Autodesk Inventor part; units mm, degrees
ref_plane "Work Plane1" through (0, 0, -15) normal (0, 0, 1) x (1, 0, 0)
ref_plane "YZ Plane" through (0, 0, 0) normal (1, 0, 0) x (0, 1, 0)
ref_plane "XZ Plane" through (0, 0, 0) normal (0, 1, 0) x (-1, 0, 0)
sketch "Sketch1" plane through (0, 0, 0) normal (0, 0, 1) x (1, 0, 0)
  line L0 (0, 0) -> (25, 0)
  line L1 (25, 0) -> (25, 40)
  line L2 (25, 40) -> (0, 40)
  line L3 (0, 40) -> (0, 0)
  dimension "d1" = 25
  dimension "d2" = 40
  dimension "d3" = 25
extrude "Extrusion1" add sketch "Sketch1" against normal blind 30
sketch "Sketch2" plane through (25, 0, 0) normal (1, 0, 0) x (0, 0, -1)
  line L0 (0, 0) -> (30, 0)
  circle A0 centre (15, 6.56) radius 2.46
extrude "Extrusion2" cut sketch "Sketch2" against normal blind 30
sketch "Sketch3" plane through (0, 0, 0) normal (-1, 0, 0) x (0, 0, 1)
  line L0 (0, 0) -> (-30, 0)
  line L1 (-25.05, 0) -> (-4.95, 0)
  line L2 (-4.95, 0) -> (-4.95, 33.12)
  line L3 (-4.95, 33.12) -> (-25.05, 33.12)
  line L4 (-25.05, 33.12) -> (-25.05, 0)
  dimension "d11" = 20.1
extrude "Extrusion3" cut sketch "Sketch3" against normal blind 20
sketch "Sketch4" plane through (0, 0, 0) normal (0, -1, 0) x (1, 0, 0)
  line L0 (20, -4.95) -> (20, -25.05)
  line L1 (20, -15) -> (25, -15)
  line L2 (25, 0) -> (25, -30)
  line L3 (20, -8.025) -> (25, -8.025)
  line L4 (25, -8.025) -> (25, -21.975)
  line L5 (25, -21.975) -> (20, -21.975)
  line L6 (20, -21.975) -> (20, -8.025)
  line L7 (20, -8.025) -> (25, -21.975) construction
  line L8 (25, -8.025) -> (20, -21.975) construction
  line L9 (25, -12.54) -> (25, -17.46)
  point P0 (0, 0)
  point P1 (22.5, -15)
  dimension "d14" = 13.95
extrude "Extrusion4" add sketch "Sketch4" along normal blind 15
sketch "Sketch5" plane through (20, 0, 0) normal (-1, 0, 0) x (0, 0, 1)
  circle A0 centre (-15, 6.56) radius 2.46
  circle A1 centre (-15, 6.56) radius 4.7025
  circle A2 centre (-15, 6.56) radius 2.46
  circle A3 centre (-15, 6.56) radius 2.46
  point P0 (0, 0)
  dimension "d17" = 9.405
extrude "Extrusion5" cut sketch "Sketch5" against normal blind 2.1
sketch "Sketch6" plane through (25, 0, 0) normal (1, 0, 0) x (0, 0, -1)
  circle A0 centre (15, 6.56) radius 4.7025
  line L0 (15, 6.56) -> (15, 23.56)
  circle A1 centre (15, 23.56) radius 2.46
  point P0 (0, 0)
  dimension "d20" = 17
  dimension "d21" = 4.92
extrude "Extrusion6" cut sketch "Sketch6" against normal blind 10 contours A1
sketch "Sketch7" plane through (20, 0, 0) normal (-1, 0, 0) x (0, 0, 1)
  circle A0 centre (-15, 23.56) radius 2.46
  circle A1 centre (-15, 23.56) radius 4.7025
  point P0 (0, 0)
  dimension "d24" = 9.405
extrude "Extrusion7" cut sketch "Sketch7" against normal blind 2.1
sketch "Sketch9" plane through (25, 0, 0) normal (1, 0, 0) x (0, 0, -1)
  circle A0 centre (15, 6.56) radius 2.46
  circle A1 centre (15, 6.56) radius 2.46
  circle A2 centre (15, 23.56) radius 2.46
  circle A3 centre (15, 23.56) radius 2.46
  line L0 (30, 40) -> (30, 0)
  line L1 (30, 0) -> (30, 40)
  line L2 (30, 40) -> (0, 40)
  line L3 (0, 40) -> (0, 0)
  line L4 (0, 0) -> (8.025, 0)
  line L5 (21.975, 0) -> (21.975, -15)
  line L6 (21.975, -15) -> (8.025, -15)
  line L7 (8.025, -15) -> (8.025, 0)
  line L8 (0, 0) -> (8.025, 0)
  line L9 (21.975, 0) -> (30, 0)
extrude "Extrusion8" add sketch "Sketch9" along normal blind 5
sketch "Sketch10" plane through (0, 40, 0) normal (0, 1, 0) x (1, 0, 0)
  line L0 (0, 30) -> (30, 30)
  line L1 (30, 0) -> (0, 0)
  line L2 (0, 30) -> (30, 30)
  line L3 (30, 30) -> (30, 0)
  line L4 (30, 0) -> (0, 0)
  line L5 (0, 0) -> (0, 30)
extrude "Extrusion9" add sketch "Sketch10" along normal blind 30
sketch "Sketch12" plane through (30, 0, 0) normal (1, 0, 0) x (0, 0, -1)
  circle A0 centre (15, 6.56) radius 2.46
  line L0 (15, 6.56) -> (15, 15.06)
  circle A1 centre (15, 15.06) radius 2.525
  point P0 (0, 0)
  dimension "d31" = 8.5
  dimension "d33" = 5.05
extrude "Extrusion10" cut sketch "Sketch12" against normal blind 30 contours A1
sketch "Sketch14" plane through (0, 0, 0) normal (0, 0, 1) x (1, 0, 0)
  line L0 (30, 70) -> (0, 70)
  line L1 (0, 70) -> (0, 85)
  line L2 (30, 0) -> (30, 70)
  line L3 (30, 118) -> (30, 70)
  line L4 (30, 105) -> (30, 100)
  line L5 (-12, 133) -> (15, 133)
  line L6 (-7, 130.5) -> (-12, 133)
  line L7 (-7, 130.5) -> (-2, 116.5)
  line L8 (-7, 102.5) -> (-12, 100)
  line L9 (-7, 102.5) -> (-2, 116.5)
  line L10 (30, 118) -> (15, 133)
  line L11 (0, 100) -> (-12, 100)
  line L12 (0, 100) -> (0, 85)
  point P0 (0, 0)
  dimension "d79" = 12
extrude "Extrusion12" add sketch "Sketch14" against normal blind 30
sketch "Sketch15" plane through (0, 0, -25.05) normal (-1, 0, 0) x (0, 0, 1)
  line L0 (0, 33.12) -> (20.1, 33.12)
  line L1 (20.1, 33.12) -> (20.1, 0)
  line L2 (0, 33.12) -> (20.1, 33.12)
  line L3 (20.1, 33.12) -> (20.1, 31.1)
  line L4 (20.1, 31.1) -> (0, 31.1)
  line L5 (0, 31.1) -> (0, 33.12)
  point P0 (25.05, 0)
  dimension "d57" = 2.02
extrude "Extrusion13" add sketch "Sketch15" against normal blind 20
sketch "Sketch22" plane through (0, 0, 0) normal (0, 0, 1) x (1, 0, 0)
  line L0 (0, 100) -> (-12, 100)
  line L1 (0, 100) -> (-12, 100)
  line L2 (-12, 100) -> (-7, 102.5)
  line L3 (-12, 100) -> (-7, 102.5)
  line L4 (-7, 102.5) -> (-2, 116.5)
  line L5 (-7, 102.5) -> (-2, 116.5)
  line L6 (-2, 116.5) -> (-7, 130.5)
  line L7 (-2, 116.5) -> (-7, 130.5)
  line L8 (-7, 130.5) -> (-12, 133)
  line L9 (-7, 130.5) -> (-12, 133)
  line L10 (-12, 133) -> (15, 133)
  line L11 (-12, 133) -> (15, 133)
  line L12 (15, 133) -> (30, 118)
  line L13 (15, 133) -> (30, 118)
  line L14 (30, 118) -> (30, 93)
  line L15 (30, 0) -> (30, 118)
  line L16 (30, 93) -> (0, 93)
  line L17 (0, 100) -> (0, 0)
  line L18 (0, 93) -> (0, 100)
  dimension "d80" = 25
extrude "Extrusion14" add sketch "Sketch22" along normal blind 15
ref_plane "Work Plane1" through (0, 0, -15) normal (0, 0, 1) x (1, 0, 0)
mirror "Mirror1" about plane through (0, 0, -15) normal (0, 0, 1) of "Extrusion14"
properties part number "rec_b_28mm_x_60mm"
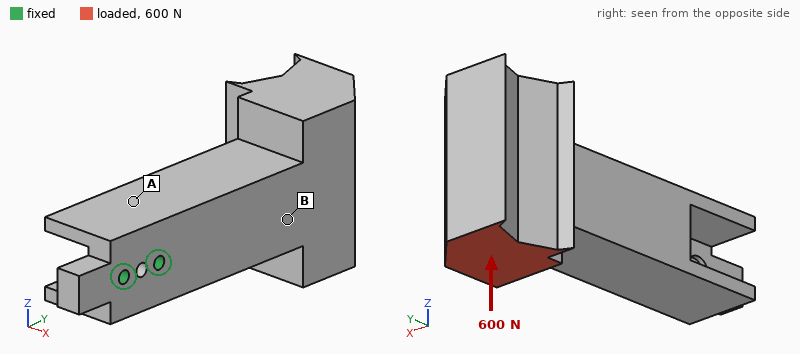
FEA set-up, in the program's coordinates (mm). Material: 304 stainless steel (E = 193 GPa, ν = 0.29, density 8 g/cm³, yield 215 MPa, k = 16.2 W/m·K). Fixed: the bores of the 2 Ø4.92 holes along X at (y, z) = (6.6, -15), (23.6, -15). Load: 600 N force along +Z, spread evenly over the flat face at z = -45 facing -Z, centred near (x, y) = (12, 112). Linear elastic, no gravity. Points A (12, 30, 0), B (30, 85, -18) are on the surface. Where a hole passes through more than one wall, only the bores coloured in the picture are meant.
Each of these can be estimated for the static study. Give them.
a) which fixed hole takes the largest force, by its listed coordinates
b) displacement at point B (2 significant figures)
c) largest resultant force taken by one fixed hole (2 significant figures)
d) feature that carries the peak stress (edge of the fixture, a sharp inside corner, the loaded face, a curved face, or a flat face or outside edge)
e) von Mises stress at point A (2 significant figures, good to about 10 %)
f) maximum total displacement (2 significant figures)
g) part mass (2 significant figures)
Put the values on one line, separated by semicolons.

(23.6, -15); 22 µm; 2.9 kN; edge of the fixture; 15 MPa; 47 µm; 1.2 kg
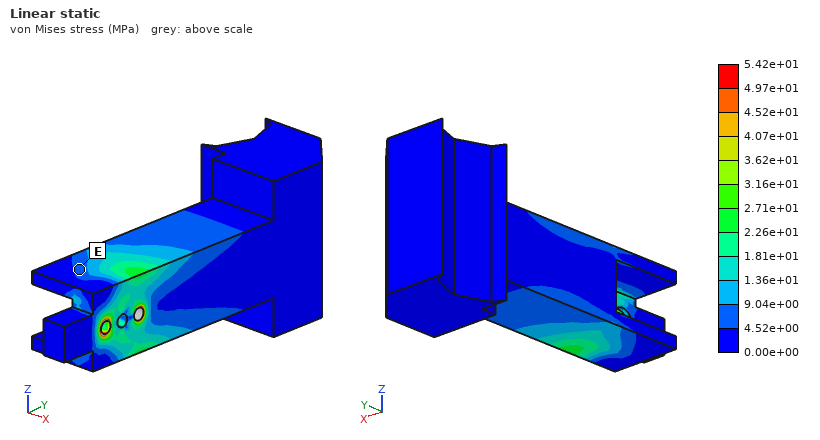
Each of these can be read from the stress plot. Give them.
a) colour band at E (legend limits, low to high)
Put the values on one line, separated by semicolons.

4.52e+00 to 9.04e+00 MPa
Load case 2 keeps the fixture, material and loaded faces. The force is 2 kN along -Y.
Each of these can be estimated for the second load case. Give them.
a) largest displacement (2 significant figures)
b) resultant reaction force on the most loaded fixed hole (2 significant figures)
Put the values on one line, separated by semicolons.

70 µm; 3.1 kN
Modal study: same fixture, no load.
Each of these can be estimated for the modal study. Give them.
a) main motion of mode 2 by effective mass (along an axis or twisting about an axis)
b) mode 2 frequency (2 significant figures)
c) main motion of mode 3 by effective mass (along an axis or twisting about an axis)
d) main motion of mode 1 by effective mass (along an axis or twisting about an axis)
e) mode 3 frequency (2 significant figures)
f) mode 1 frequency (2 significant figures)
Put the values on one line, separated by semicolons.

along Z; 770 Hz; twisting about Y; along X; 1800 Hz; 670 Hz
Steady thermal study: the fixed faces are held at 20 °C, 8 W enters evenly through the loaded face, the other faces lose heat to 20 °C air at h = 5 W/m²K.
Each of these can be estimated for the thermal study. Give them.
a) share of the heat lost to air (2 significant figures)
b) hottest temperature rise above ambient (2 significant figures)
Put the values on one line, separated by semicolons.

38 %; 49 K
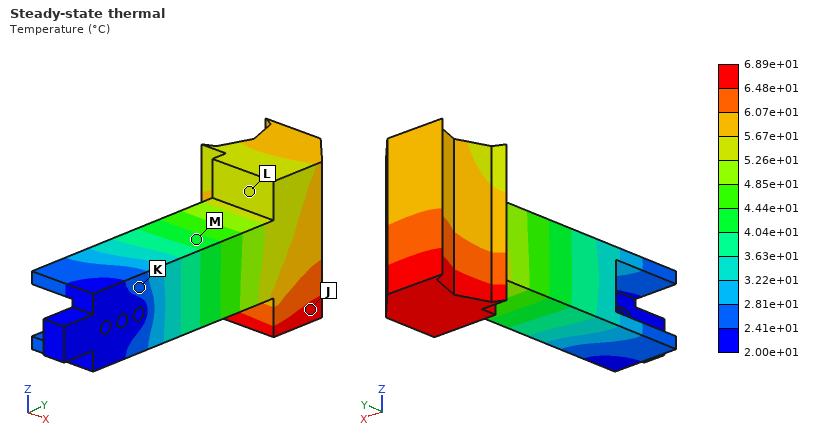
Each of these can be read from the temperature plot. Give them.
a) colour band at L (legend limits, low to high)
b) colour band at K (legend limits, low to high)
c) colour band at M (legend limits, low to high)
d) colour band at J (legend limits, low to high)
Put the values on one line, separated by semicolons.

5.26e+01 to 5.67e+01 °C; 2.41e+01 to 2.81e+01 °C; 4.04e+01 to 4.44e+01 °C; 6.48e+01 to 6.89e+01 °C
